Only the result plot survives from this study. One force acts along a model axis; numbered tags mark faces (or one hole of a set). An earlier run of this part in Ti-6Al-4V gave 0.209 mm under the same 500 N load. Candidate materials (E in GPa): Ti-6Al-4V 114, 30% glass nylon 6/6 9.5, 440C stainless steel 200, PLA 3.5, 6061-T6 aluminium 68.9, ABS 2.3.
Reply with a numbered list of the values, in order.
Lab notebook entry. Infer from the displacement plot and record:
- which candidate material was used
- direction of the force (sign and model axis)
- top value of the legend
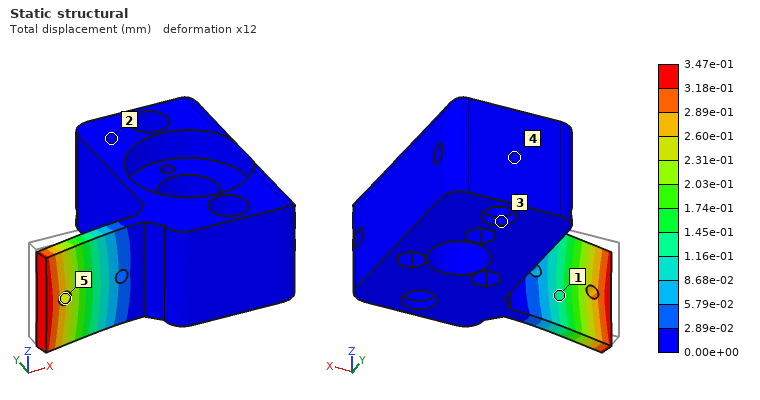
1. 6061-T6 aluminium
2. -Y
3. 3.47e-01 mm
